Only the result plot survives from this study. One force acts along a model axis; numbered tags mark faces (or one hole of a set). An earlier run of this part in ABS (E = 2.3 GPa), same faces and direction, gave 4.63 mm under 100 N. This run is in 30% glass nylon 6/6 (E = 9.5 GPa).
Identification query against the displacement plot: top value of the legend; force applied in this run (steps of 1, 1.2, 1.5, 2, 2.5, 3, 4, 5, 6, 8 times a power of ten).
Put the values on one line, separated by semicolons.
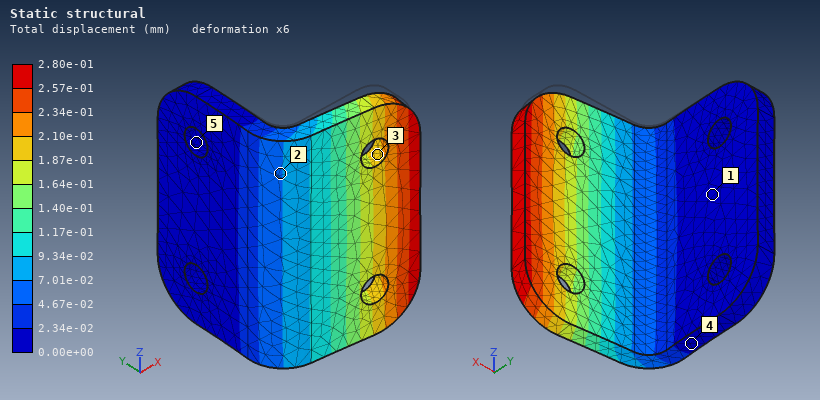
2.80e-01 mm; 25 N
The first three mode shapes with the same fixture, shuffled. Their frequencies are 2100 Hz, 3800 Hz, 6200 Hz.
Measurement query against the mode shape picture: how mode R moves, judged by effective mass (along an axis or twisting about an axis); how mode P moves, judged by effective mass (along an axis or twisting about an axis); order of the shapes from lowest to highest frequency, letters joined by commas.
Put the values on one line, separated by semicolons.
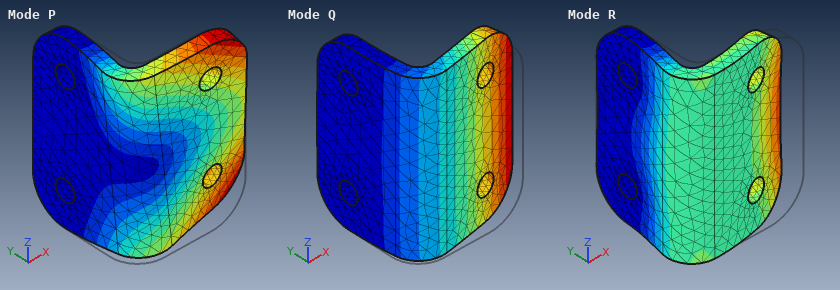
along X; along Z; Q, P, R
